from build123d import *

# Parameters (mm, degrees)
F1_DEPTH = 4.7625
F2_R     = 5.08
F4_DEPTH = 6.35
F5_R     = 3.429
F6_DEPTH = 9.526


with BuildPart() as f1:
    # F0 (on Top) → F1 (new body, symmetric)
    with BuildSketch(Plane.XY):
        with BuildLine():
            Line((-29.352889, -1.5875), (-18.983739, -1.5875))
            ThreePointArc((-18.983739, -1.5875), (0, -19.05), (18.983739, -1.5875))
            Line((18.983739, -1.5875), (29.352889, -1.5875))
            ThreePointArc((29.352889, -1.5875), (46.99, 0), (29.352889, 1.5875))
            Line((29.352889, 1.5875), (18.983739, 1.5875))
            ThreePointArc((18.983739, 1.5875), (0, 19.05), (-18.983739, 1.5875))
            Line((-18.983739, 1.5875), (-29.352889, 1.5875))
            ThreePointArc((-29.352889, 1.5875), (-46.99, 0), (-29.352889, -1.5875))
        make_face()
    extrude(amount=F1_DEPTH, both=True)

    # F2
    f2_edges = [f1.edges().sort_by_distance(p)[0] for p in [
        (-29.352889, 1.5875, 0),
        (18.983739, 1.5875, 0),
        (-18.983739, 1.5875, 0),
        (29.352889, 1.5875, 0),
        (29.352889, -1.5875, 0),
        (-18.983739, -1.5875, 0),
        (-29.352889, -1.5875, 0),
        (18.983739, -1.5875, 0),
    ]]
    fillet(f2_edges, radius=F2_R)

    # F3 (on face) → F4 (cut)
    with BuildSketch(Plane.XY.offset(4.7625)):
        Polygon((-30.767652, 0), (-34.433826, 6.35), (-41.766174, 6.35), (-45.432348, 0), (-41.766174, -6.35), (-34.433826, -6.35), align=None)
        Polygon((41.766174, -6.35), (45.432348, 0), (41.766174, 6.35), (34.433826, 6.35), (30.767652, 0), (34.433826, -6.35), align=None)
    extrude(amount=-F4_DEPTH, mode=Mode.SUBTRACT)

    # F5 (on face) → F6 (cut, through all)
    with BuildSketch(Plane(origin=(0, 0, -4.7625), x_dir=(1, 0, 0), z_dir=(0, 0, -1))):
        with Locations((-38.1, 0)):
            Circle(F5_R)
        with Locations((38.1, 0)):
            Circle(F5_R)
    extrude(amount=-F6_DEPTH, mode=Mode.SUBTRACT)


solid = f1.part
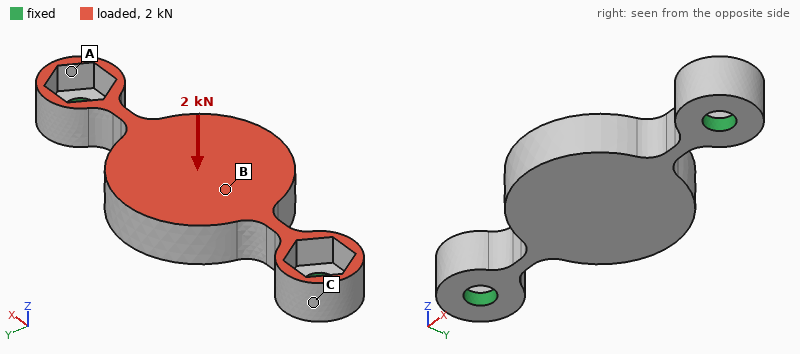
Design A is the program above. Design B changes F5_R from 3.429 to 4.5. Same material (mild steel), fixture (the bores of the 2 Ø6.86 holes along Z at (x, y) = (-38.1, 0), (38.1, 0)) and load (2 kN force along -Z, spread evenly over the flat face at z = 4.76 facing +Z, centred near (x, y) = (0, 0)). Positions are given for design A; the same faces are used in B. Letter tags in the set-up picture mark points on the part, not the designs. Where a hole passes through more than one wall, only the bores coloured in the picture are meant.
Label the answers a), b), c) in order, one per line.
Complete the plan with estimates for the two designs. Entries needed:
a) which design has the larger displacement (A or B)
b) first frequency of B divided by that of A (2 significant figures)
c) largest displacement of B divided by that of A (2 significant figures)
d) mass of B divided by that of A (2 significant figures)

a) A
b) 1.0
c) 0.89
d) 0.99
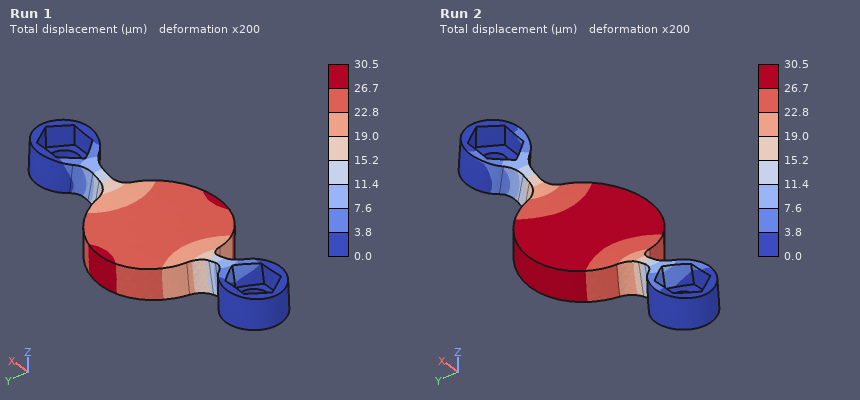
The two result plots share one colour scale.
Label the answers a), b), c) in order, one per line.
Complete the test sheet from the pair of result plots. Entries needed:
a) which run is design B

a) Run 1
